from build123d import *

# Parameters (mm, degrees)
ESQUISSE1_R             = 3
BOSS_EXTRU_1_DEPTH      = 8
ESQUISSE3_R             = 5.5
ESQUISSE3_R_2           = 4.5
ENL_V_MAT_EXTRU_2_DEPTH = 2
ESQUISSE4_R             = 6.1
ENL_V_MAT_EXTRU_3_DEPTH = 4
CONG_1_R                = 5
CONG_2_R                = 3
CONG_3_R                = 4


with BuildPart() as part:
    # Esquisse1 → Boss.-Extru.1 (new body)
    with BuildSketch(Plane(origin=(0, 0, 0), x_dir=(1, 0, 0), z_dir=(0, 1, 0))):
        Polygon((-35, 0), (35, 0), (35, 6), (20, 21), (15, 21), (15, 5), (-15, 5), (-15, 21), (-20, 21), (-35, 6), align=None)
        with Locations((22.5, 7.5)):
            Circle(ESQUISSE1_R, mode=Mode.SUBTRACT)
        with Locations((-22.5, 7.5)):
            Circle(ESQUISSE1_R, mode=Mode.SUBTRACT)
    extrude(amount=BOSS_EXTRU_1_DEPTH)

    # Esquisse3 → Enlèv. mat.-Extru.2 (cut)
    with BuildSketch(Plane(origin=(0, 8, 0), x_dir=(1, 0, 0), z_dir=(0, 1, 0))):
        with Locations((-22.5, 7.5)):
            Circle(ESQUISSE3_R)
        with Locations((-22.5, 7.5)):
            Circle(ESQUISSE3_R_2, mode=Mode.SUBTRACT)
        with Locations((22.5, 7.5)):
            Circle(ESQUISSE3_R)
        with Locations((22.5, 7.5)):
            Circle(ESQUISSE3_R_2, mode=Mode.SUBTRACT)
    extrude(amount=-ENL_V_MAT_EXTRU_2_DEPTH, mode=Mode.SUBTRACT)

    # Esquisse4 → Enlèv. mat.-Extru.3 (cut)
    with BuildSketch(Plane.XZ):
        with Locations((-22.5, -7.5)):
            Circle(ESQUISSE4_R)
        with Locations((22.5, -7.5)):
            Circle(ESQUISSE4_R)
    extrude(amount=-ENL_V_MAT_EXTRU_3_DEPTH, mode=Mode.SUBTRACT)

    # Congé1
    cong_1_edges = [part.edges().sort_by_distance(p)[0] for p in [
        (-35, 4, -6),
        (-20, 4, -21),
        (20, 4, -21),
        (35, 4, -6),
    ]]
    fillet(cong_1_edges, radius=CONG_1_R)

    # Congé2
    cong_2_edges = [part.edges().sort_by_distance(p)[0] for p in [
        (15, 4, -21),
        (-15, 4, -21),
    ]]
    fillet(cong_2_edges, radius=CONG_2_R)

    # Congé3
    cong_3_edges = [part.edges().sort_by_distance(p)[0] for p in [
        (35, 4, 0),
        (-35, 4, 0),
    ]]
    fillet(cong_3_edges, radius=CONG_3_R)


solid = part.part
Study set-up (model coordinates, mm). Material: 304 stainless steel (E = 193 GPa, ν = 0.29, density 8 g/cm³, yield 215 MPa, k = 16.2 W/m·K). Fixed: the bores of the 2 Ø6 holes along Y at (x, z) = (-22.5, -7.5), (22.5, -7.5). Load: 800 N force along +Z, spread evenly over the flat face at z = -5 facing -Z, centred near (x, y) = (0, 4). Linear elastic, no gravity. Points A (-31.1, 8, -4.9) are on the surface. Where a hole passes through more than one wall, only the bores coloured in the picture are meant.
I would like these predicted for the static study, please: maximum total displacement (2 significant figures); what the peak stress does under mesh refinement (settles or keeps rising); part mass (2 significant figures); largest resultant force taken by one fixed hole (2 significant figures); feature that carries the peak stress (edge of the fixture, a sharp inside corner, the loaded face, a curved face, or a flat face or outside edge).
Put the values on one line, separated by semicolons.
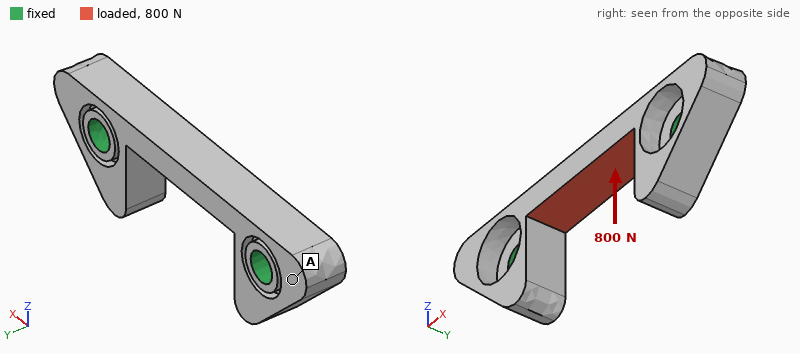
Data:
12 µm; keeps rising; 38 g; 460 N; edge of the fixture
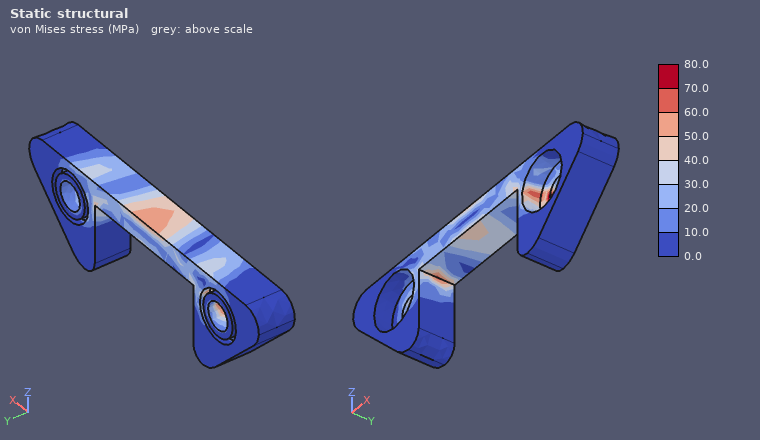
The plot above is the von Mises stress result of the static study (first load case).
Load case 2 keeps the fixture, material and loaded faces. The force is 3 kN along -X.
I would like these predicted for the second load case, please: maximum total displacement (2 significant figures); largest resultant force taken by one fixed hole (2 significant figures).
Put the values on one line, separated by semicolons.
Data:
6.5 µm; 1.5 kN
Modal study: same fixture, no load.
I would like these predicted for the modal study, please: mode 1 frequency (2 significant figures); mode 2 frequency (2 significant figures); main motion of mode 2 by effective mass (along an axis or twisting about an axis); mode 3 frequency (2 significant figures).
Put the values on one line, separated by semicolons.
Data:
12 kHz; 15 kHz; along Z; 16 kHz
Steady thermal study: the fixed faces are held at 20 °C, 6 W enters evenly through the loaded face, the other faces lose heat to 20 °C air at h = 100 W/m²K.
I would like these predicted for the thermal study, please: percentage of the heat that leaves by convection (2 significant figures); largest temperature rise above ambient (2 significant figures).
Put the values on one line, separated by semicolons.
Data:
50 %; 46 K
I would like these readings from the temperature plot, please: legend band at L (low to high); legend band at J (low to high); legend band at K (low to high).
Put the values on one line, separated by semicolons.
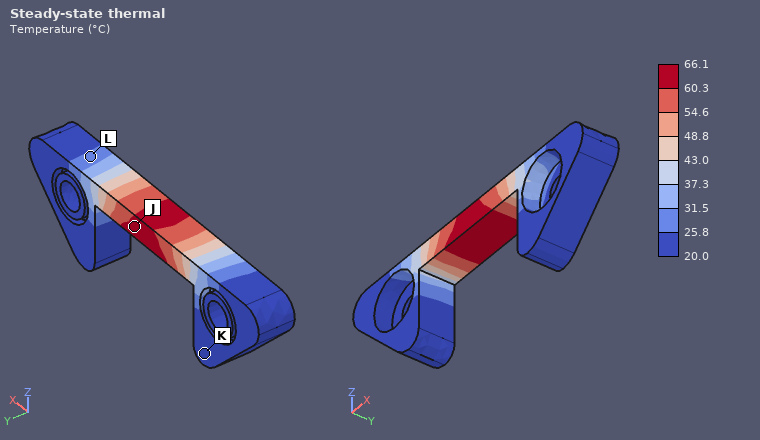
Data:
25.8 to 31.5 °C; 60.3 to 66.1 °C; 20.0 to 25.8 °C
